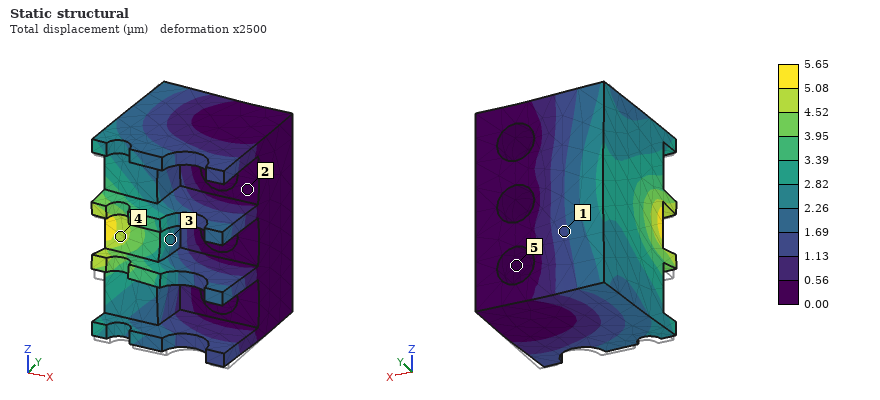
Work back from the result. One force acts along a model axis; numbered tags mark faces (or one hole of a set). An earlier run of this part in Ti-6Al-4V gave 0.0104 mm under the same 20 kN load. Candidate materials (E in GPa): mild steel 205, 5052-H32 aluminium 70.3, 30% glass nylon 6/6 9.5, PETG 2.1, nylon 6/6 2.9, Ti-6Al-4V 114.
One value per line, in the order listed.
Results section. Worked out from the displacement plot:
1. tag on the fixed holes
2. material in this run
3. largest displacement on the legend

5
mild steel
5.65 µm
